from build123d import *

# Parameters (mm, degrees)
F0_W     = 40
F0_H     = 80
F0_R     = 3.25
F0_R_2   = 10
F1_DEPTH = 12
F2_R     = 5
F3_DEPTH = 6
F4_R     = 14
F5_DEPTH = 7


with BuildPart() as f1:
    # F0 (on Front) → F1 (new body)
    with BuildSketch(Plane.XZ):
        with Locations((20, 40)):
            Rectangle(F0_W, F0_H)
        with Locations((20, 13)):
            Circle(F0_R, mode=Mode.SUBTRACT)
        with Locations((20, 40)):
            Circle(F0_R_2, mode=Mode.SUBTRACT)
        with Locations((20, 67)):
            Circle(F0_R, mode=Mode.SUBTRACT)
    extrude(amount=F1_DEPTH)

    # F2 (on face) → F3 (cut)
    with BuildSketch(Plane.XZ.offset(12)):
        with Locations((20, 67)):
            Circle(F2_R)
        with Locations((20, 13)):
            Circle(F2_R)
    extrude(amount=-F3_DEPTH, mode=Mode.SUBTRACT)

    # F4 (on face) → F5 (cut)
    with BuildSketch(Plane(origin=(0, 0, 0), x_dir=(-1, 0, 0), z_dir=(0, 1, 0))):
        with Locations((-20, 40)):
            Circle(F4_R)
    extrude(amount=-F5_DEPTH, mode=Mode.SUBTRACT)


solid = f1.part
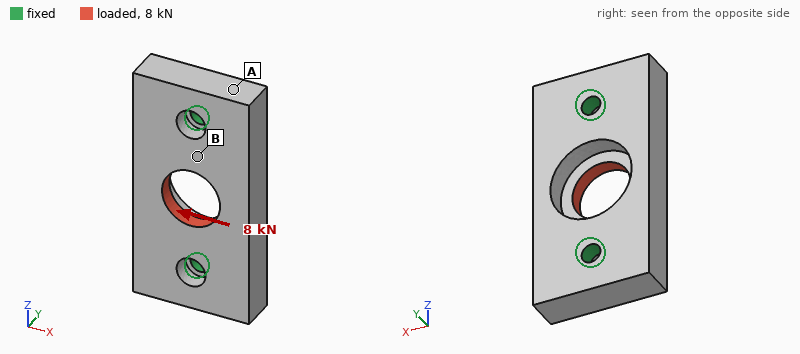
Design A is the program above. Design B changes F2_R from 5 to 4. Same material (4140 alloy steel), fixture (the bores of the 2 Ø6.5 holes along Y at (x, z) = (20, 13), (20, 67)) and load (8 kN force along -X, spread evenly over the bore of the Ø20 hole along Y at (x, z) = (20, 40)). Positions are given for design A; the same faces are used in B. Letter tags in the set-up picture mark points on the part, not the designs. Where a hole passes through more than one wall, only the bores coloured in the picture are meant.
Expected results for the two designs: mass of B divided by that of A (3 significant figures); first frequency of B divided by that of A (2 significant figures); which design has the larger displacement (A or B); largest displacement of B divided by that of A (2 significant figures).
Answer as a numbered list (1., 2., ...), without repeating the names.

1. 1.01
2. 1.0
3. A
4. 0.91
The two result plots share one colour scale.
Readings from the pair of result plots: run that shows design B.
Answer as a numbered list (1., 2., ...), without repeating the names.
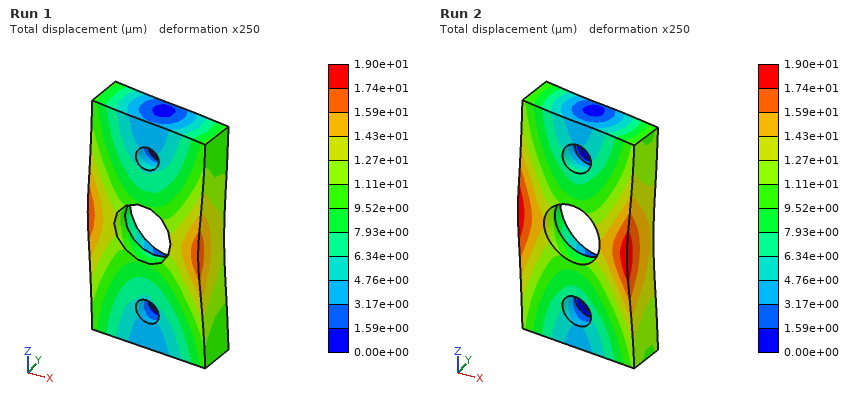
1. Run 1
